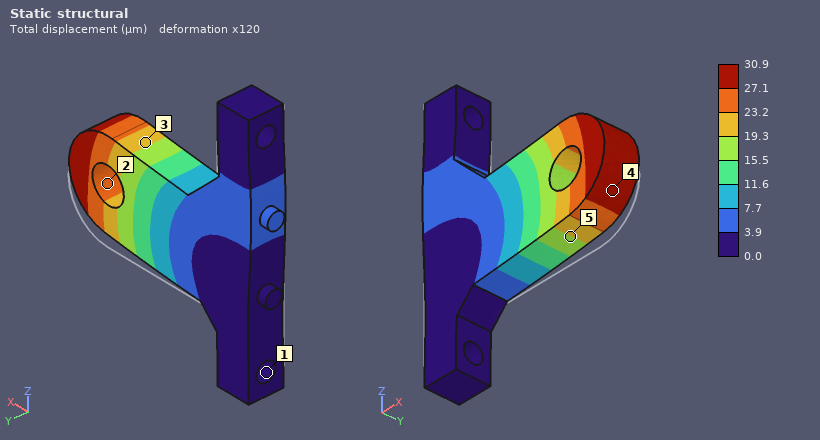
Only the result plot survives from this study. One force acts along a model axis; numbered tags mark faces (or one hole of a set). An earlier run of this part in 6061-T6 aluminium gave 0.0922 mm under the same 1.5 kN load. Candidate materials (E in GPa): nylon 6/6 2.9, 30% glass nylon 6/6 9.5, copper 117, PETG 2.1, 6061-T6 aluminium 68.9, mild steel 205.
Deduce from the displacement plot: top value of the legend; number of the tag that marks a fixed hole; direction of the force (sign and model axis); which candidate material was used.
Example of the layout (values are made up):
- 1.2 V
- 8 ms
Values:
- 30.9 µm
- 1
- +Z
- mild steel
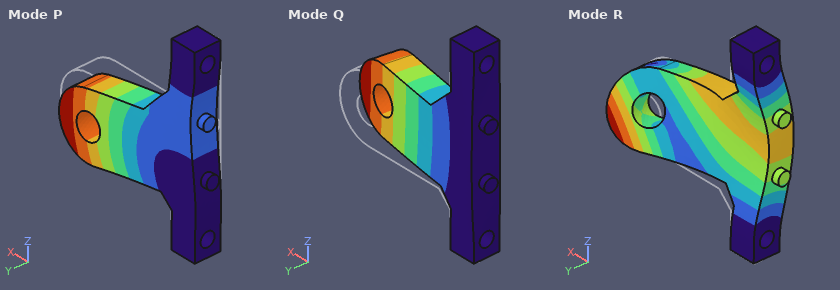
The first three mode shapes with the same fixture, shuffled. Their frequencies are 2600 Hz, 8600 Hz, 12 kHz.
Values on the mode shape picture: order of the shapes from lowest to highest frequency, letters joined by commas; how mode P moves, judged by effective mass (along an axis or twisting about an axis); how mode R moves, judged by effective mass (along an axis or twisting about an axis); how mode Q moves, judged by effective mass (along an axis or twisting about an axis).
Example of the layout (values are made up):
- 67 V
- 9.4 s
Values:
- Q, P, R
- along Z
- along Y
- along Y
